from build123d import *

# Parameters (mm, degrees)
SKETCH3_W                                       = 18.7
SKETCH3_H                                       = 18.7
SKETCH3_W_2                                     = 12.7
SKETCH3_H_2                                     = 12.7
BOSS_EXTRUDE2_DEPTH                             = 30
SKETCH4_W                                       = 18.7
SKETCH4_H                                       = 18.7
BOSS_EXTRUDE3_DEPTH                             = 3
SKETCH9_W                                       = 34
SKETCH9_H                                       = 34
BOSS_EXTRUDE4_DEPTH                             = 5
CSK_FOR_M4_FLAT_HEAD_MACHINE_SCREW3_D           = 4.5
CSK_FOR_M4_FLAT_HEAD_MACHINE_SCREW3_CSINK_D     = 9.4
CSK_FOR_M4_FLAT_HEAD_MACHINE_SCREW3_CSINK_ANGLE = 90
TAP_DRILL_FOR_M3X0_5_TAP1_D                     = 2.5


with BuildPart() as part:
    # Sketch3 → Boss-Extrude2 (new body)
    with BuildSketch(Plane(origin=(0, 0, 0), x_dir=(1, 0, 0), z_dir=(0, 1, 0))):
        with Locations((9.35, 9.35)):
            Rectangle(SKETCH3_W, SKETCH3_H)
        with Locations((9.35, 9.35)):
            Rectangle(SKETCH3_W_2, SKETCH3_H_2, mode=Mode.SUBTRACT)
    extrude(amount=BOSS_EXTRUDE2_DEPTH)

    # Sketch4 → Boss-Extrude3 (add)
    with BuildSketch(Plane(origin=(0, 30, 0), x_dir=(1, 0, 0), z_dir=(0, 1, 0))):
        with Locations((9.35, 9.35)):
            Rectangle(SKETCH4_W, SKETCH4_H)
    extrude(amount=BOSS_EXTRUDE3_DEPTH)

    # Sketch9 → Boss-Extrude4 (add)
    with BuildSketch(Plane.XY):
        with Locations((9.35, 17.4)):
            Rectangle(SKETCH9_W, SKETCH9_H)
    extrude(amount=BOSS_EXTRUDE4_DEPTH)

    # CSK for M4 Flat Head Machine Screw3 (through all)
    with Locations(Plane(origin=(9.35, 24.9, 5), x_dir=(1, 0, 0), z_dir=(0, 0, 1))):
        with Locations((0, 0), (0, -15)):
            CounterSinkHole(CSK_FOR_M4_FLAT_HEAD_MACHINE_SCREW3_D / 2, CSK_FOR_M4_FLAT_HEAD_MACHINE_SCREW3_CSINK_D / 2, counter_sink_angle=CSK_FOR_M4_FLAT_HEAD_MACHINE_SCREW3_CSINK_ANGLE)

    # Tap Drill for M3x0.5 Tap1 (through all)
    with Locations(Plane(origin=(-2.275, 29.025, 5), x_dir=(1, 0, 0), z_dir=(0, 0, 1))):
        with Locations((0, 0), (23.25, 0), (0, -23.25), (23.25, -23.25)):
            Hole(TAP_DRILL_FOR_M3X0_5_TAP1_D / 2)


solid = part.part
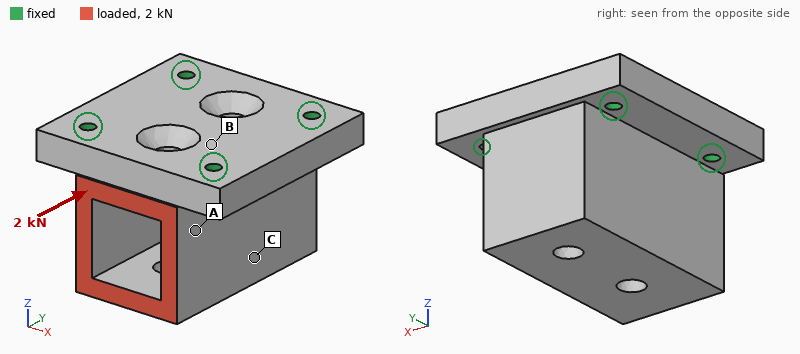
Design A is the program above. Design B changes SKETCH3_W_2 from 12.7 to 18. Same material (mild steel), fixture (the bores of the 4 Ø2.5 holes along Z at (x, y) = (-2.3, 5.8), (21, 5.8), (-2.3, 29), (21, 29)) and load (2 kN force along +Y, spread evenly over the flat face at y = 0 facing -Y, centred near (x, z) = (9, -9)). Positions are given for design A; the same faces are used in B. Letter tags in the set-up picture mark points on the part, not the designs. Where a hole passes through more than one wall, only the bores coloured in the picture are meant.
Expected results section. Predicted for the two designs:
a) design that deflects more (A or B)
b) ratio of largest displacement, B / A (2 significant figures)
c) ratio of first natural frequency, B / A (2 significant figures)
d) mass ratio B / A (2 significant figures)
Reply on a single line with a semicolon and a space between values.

B; 2.8; 0.50; 0.83
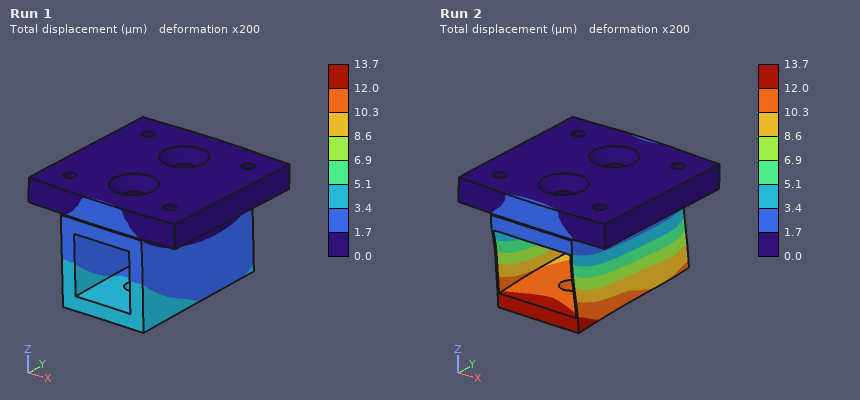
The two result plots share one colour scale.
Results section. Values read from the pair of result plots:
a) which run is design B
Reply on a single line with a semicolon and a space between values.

Run 2
